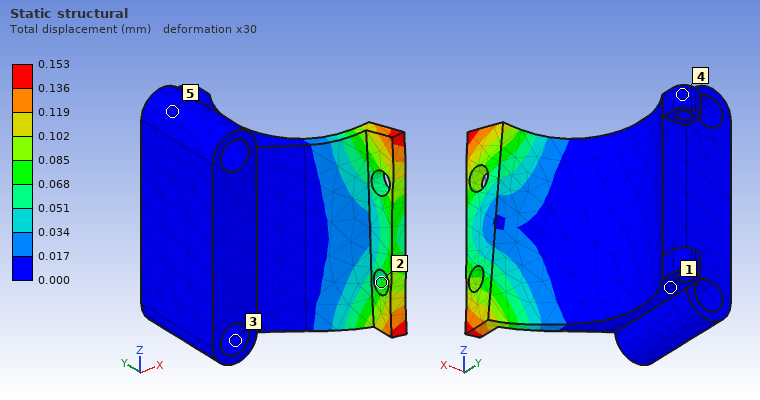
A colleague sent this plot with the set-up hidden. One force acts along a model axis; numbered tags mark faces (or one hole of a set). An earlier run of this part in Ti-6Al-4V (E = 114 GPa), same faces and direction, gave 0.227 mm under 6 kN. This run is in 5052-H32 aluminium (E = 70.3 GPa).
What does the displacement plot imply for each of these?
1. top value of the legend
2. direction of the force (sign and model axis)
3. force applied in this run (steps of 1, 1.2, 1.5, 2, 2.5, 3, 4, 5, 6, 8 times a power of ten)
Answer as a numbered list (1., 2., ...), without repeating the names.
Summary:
1. 0.153 mm
2. +Z
3. 2.5 kN
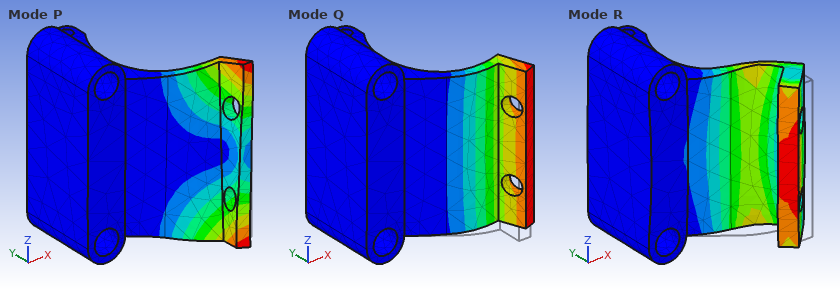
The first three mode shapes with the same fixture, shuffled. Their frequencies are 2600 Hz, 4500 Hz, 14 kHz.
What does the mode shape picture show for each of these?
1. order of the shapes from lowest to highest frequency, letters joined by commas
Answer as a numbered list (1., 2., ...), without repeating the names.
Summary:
1. Q, P, R
